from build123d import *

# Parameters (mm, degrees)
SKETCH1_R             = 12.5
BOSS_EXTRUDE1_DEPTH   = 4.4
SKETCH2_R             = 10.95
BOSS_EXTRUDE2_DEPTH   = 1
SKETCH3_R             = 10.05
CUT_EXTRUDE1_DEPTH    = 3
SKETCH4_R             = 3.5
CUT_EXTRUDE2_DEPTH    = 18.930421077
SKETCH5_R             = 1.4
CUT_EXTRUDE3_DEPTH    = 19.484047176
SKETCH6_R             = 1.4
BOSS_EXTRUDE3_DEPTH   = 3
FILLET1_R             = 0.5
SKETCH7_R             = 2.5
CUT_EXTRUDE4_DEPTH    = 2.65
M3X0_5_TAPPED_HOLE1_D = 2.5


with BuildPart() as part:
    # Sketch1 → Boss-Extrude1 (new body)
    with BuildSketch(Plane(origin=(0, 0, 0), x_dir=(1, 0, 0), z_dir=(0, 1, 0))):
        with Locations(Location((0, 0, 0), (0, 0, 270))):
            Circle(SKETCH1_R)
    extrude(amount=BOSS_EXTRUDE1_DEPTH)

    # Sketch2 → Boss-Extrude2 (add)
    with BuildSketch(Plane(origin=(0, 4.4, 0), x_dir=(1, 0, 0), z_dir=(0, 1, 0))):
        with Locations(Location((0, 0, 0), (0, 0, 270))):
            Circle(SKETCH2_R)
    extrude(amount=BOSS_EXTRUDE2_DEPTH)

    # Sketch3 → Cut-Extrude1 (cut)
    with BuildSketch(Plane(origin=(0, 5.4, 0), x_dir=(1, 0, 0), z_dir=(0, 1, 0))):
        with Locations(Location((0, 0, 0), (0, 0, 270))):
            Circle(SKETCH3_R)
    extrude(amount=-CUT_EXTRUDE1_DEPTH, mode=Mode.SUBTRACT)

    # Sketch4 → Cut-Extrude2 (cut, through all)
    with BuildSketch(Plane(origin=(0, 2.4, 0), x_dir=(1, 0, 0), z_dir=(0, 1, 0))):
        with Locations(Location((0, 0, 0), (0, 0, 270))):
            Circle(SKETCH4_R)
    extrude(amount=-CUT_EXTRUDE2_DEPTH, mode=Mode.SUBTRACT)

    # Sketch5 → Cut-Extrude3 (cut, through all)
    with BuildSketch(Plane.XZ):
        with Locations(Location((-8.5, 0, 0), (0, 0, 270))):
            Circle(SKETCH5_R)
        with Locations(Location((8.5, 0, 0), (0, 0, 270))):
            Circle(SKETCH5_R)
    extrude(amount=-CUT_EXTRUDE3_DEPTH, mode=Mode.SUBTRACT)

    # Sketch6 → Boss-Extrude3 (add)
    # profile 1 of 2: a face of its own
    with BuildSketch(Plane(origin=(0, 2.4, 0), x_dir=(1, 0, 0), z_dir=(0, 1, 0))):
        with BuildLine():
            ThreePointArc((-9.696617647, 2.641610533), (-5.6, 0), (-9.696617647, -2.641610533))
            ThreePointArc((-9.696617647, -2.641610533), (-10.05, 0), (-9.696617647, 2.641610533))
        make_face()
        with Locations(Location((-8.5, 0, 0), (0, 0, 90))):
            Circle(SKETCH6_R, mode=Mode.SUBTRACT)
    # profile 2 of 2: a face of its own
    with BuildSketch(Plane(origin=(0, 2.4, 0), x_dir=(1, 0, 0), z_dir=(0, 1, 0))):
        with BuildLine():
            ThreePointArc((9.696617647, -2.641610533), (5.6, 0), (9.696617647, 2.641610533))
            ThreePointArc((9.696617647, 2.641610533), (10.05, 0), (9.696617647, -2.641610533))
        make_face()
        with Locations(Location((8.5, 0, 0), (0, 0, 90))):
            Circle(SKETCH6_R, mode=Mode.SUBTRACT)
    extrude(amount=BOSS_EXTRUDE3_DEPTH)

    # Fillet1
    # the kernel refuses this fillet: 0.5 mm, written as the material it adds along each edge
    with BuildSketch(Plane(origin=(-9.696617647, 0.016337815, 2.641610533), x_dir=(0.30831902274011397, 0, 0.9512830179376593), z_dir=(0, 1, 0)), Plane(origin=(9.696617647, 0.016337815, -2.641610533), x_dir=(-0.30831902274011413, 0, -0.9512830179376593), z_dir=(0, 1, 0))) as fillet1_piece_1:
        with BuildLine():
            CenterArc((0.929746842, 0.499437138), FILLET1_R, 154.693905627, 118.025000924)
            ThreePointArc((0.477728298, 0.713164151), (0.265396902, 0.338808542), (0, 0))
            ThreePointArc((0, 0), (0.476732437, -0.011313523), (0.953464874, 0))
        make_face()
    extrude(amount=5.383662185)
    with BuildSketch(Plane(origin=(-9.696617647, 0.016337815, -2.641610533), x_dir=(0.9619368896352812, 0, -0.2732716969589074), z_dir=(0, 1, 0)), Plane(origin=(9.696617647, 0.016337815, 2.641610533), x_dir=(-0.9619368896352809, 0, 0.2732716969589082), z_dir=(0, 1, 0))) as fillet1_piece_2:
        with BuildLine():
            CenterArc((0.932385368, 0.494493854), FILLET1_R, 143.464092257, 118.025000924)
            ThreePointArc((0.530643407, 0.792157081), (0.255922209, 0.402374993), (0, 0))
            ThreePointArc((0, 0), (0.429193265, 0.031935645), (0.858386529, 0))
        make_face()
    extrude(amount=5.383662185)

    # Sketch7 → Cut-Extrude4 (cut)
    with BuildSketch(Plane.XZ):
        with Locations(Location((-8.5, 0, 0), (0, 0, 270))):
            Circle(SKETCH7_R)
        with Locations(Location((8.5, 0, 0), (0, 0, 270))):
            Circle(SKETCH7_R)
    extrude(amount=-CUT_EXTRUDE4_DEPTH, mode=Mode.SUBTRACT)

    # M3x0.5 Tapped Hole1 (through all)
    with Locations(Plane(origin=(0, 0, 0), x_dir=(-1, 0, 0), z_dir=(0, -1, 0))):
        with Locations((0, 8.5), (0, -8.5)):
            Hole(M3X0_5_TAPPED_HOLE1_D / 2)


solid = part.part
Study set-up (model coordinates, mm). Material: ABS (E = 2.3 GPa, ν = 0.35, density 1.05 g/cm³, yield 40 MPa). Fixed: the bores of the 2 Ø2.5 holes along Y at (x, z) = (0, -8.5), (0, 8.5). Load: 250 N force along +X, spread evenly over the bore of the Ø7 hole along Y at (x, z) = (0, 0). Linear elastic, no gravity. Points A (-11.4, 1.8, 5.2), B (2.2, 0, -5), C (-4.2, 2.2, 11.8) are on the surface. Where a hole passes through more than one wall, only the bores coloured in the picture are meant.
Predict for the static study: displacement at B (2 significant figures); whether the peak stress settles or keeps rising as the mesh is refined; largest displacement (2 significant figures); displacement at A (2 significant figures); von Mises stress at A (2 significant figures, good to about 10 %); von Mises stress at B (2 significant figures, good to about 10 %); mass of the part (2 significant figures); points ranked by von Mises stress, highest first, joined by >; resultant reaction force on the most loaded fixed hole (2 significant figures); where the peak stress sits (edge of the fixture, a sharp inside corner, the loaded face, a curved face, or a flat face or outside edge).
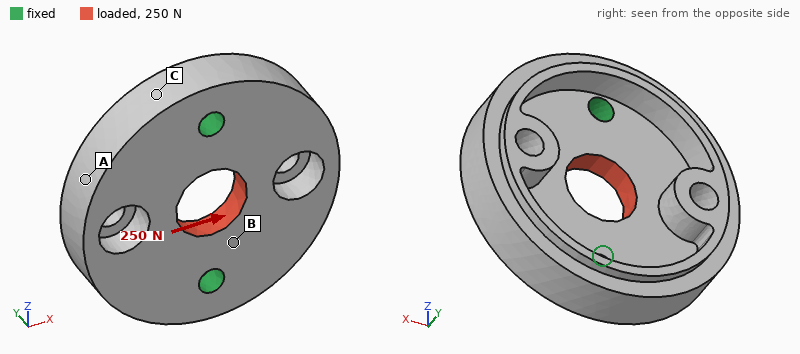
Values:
16 µm
keeps rising
37 µm
17 µm
3.2 MPa
5.1 MPa
1.5 g
B > A > C
130 N
edge of the fixture
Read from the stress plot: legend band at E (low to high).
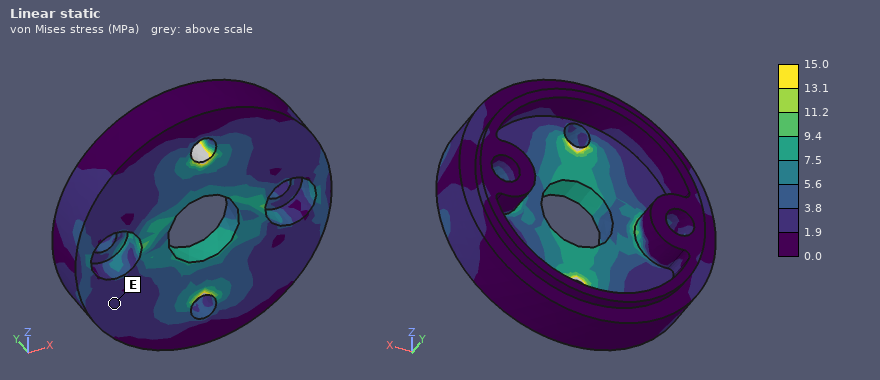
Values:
1.9 to 3.8 MPa
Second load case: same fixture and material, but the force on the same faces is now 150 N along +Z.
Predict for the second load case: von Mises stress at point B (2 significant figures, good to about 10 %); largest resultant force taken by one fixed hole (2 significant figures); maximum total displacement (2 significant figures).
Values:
3.9 MPa
75 N
14 µm
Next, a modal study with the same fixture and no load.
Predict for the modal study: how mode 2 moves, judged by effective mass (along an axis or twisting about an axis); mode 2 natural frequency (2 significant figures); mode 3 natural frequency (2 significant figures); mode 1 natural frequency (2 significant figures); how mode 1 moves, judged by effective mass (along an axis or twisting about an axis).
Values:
along Y
5000 Hz
8700 Hz
3800 Hz
twisting about Z
